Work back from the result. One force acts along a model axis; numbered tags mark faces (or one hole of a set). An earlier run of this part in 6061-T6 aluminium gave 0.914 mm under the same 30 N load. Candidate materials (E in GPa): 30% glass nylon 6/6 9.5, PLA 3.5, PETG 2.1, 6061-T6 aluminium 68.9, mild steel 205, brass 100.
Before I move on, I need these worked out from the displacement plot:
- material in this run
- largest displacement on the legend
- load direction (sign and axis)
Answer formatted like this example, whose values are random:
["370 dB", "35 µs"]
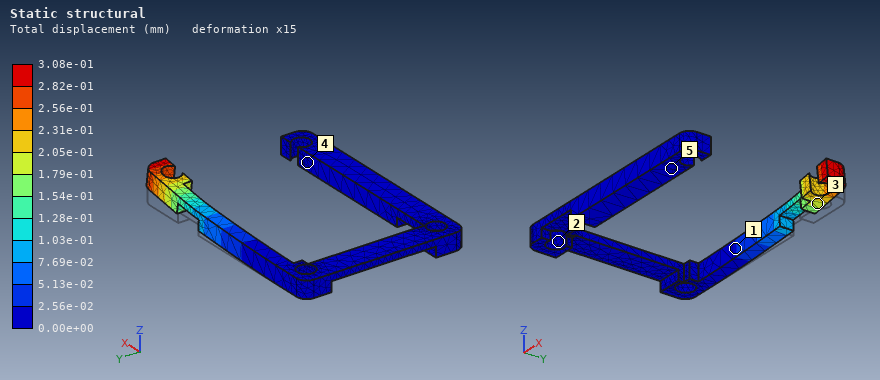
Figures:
["mild steel", "3.08e-01 mm", "+Z"]
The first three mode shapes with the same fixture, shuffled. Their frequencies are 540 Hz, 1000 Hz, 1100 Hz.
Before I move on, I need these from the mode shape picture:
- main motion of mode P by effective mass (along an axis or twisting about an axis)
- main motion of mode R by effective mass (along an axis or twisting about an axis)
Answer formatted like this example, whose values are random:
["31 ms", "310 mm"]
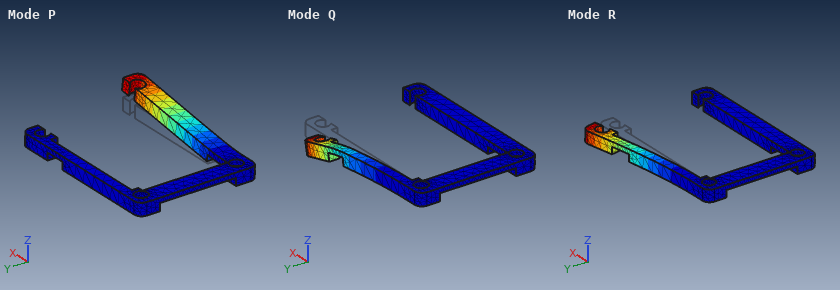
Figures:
["along Z", "along Y"]
